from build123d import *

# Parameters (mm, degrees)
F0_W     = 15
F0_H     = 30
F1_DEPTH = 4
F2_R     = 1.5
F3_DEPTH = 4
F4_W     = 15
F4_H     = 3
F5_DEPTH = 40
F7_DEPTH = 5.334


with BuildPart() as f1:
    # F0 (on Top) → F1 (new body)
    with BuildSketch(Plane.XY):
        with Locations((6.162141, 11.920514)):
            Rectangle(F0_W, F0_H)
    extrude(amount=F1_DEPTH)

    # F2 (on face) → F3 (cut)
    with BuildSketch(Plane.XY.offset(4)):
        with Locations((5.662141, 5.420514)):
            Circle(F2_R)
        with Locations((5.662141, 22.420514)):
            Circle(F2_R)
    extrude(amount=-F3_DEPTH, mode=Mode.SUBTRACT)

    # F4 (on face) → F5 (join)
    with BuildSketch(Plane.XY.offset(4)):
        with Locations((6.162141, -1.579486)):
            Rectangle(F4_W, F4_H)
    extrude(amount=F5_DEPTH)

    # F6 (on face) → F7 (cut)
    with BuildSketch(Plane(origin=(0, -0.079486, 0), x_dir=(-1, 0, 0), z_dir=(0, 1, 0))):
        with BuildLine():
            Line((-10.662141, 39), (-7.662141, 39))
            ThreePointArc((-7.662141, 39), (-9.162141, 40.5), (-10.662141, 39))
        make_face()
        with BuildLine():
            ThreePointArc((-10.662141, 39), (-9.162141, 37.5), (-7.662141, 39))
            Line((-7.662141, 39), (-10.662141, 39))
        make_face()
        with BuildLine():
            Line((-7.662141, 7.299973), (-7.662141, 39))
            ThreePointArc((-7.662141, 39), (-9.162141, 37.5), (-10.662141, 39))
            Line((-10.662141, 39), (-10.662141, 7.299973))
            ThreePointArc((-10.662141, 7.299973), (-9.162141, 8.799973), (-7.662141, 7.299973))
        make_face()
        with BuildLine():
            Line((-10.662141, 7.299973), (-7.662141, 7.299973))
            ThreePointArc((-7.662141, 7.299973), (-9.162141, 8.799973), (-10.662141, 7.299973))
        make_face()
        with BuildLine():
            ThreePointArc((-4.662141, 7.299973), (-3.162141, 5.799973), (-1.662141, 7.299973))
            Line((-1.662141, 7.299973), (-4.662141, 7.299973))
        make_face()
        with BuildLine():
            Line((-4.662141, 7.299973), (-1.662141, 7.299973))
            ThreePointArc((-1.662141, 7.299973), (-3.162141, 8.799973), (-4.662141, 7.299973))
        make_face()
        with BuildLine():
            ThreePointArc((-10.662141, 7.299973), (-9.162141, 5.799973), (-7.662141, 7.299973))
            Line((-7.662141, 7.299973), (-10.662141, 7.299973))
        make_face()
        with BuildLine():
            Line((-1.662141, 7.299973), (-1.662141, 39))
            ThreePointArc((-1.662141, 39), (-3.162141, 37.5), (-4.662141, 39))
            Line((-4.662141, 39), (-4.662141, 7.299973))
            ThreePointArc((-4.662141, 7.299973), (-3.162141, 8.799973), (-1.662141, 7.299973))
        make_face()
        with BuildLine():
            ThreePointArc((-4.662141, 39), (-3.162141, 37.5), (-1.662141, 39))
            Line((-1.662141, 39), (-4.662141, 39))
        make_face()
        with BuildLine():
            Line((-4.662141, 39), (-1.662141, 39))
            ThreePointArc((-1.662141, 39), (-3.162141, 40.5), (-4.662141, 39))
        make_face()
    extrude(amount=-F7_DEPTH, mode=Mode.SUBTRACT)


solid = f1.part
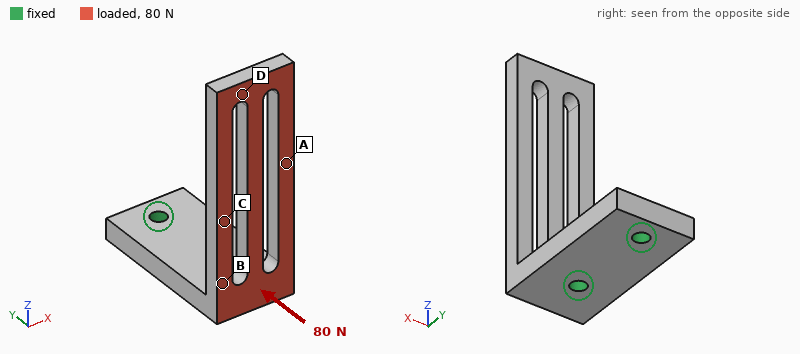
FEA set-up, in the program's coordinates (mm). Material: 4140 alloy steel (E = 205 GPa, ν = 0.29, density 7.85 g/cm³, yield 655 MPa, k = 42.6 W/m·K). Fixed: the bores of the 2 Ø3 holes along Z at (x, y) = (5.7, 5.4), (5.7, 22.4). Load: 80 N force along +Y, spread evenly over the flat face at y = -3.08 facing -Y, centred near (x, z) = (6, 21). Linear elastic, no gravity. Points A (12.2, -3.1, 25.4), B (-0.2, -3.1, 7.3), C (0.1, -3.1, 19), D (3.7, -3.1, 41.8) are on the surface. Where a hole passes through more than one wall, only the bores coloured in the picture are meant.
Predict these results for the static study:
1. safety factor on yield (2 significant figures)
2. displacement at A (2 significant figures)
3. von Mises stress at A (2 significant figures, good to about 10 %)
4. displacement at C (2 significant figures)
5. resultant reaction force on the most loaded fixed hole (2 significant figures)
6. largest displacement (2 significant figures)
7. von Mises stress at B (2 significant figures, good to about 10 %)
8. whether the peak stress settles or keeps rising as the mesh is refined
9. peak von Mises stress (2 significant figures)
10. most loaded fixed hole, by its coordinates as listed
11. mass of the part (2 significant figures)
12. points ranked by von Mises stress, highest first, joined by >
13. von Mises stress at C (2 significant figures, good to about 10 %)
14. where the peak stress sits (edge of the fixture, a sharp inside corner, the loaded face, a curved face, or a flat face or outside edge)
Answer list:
5.5
0.073 mm
25 MPa
0.043 mm
76 N
0.17 mm
83 MPa
settles
120 MPa
(5.7, 5.4)
23 g
B > C > A > D
43 MPa
the loaded face
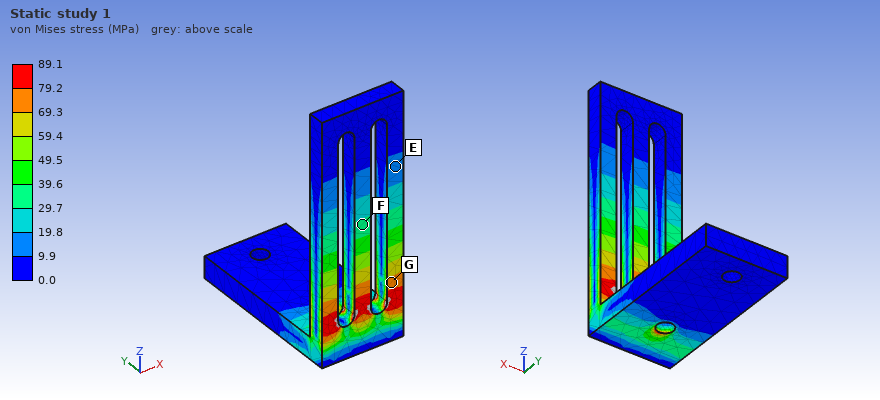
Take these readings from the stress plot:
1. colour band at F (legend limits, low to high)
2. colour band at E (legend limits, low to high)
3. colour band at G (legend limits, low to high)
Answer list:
29.7 to 39.6 MPa
9.9 to 19.8 MPa
69.3 to 79.2 MPa
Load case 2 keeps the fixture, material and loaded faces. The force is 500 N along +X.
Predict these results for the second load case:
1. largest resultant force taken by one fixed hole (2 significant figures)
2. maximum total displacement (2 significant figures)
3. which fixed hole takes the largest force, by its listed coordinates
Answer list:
670 N
0.36 mm
(5.7, 5.4)
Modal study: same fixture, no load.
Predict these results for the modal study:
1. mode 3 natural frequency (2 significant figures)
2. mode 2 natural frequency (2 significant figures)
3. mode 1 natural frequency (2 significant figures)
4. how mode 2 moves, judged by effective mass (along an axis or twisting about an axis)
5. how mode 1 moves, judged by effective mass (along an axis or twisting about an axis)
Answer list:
4800 Hz
2100 Hz
1300 Hz
along X
along Y
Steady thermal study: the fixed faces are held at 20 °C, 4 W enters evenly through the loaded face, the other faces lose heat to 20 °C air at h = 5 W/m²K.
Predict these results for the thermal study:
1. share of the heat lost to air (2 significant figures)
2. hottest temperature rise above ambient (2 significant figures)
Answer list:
7.0 %
67 K
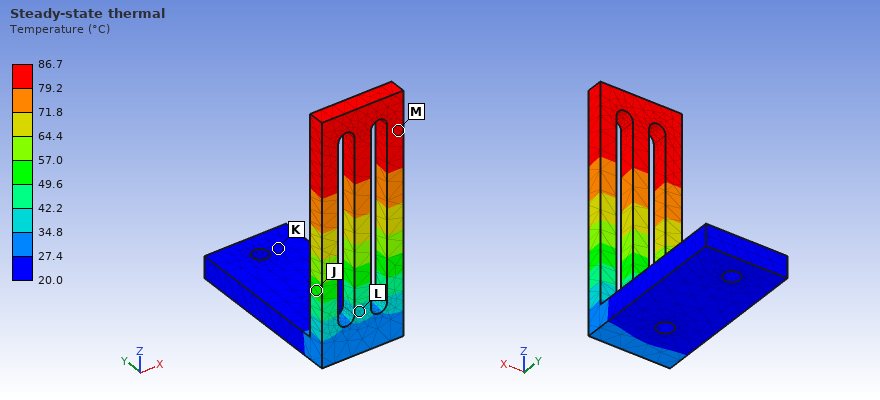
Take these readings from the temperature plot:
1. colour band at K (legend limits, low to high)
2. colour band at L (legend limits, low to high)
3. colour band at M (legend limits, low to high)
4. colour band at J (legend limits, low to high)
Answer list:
20.0 to 27.4 °C
34.8 to 42.2 °C
79.2 to 86.7 °C
49.6 to 57.0 °C
